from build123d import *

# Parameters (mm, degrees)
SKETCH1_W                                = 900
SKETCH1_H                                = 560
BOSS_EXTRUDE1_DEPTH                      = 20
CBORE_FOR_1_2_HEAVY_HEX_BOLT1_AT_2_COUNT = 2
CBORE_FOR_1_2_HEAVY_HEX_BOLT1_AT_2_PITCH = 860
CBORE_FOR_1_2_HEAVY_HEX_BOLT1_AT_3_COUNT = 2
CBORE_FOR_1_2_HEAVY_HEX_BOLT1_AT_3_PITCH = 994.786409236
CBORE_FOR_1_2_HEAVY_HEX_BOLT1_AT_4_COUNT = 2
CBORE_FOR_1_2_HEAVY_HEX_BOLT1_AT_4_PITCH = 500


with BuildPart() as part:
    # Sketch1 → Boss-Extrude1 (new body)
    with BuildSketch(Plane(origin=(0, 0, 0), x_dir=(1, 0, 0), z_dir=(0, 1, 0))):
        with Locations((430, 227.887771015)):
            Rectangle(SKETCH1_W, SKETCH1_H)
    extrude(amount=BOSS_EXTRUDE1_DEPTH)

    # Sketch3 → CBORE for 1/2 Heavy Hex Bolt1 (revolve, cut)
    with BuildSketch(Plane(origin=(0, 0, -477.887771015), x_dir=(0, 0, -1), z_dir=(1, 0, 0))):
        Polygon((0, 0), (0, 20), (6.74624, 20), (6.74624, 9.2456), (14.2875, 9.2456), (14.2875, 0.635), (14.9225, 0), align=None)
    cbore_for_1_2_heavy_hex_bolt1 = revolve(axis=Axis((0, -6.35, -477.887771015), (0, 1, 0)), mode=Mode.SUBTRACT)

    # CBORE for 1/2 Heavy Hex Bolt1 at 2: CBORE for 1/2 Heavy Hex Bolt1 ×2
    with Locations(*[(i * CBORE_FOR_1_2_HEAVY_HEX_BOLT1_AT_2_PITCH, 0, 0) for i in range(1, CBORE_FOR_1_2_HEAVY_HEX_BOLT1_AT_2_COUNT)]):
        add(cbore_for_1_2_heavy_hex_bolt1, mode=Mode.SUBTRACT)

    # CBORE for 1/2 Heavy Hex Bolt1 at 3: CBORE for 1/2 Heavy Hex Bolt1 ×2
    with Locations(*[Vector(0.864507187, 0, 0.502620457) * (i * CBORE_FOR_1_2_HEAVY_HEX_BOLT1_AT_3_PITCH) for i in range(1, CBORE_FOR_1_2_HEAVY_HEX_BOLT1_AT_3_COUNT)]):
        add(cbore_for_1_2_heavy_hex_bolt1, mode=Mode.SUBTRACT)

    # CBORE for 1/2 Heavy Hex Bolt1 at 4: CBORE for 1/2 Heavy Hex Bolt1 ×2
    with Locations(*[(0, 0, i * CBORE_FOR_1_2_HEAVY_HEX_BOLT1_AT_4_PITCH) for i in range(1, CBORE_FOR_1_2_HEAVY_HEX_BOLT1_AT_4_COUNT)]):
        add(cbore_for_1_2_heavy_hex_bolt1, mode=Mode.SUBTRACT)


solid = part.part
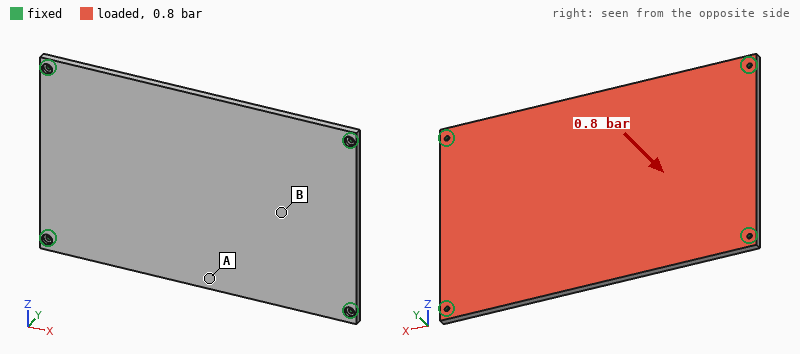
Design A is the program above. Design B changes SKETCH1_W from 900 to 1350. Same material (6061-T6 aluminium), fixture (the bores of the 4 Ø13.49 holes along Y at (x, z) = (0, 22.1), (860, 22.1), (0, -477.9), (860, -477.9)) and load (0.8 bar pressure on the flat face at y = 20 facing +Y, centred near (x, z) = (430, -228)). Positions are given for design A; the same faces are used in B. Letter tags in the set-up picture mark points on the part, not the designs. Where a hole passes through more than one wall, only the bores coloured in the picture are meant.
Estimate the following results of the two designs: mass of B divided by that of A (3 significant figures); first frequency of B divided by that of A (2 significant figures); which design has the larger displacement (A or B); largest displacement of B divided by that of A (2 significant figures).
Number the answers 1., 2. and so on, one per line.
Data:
1. 1.50
2. 0.98
3. A
4. 0.75
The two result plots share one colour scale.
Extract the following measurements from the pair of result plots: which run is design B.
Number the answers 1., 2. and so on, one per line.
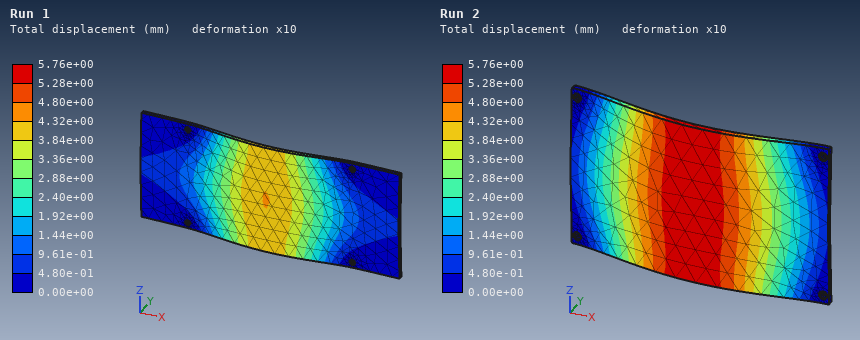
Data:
1. Run 1
